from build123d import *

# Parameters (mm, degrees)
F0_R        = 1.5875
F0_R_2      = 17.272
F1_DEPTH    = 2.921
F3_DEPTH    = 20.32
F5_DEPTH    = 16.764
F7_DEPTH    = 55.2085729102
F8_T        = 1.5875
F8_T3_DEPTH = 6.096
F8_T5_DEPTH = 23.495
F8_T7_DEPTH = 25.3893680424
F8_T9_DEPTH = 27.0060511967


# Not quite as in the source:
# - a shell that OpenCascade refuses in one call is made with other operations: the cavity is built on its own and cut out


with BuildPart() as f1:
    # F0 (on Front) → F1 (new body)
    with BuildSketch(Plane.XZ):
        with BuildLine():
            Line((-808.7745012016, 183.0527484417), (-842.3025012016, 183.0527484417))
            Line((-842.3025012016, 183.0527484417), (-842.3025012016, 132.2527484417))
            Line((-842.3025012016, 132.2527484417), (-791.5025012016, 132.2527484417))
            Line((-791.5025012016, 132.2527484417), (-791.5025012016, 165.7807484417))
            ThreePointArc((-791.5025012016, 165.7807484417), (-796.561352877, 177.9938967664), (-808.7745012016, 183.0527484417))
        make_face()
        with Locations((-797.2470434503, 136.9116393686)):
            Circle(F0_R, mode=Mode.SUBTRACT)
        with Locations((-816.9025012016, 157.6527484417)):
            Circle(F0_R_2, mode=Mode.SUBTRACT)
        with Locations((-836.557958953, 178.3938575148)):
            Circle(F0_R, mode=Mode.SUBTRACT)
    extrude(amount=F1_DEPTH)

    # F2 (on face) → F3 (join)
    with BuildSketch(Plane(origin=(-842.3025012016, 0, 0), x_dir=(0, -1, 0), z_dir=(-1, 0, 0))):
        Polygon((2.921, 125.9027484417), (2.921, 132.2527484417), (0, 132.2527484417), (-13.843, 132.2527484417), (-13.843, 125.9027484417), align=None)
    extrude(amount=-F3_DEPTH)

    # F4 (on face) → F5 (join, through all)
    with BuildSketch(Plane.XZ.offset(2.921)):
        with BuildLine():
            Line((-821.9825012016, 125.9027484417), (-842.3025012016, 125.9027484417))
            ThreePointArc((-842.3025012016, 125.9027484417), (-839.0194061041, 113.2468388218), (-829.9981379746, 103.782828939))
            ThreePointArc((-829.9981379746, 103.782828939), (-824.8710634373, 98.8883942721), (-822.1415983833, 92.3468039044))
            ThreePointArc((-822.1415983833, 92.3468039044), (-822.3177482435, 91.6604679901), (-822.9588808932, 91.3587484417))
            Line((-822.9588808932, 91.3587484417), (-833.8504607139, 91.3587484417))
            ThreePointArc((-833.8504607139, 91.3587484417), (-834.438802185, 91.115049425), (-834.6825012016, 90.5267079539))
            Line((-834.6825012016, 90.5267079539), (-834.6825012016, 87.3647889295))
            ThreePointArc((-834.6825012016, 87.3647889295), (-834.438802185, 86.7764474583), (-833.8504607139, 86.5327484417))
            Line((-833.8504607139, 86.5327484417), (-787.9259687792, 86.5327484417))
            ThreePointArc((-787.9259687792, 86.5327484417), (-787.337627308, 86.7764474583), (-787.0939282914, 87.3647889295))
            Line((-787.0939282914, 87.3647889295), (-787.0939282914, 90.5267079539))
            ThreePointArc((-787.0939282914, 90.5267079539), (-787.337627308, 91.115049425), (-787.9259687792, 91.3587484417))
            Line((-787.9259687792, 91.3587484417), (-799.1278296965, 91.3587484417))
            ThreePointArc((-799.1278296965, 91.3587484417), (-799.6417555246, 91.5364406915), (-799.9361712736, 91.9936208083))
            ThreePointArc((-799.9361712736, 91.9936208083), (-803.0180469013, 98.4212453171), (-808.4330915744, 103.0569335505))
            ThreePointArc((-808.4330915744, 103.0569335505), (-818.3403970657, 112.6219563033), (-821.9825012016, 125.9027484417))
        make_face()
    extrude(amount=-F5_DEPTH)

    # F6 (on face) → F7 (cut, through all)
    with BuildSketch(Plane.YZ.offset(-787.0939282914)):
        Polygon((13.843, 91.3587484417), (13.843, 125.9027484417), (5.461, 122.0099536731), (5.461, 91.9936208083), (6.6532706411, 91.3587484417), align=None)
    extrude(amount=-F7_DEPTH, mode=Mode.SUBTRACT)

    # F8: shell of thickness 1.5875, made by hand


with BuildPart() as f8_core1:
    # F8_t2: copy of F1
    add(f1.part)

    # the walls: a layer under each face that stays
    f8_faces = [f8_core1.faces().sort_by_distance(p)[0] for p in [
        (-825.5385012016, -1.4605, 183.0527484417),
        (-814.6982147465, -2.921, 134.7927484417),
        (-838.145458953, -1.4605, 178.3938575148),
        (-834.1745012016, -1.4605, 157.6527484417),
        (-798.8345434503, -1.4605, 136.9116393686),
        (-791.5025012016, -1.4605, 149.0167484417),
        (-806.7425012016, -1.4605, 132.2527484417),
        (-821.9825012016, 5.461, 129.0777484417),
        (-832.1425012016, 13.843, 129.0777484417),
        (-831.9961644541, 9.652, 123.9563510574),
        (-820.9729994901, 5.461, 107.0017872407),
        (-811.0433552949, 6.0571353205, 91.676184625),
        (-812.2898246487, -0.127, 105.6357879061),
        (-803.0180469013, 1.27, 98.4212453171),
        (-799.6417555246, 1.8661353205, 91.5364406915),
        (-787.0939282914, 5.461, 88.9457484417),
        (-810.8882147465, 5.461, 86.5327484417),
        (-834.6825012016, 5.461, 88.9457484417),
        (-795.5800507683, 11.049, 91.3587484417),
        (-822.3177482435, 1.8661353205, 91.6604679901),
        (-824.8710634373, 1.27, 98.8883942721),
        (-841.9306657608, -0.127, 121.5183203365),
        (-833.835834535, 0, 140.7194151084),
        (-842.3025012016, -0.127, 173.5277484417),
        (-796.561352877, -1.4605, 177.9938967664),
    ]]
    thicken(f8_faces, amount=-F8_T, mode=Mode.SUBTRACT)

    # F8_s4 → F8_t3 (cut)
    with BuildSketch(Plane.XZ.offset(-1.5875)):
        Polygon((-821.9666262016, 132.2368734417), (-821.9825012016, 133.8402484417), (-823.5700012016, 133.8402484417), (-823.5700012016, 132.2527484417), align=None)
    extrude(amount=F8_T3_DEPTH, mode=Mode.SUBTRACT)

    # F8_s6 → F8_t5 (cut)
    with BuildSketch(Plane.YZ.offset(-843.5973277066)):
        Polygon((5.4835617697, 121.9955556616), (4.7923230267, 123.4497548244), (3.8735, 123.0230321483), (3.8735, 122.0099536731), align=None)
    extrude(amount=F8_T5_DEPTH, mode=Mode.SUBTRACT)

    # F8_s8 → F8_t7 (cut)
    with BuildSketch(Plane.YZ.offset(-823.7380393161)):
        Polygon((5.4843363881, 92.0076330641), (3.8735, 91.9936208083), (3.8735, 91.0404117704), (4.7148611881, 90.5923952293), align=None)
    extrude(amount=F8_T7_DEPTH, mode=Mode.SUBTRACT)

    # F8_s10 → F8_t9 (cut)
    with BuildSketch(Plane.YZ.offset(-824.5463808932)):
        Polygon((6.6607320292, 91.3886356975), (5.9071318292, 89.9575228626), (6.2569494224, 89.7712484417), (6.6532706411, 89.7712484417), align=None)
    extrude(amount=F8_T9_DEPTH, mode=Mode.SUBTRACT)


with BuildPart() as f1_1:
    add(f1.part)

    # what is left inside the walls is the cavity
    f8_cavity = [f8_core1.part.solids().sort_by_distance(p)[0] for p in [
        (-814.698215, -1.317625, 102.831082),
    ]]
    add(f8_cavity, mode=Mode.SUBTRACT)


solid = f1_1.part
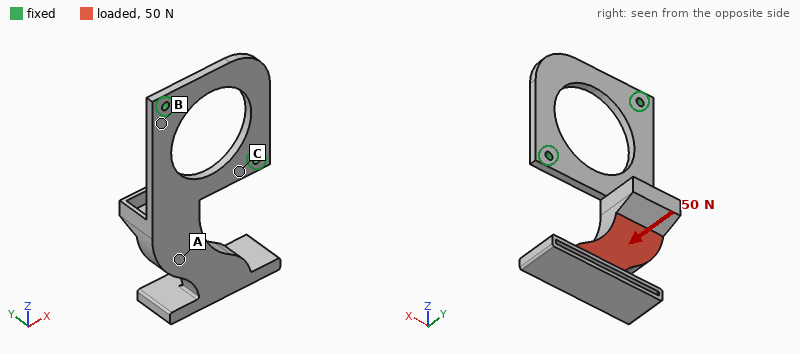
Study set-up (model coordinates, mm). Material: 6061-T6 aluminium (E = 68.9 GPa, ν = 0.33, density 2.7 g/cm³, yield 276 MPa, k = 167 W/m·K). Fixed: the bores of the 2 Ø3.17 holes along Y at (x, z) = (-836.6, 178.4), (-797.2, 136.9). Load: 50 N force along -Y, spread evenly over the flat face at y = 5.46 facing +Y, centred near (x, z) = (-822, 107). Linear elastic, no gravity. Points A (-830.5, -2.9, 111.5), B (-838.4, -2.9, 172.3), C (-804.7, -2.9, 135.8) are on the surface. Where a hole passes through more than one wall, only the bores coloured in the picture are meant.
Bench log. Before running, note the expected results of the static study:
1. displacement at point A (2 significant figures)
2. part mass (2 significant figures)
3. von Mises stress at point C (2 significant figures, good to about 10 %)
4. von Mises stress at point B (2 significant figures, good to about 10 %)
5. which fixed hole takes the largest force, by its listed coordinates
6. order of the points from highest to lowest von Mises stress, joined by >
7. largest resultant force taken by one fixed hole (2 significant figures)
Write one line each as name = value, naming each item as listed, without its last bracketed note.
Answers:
displacement at point A = 0.63 mm
part mass = 30 g
von Mises stress at point C = 75 MPa
von Mises stress at point B = 25 MPa
which fixed hole takes the largest force, by its listed coordinates = (-797.2, 136.9)
order of the points from highest to lowest von Mises stress, joined by > = C > B > A
largest resultant force taken by one fixed hole = 60 N
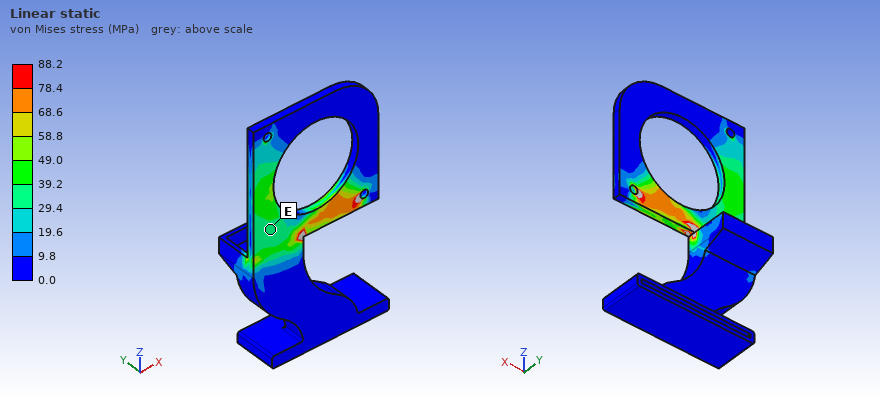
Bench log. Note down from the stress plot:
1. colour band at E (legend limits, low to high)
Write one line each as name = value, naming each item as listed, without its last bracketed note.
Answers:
colour band at E = 29.4 to 39.2 MPa
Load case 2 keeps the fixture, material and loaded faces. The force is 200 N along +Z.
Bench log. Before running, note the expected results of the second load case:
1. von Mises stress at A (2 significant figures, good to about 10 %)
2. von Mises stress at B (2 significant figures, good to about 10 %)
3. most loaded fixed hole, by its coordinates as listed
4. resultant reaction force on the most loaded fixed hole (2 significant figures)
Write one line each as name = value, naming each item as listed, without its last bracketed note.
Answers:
von Mises stress at A = 5.1 MPa
von Mises stress at B = 9.4 MPa
most loaded fixed hole, by its coordinates as listed = (-836.6, 178.4)
resultant reaction force on the most loaded fixed hole = 120 N
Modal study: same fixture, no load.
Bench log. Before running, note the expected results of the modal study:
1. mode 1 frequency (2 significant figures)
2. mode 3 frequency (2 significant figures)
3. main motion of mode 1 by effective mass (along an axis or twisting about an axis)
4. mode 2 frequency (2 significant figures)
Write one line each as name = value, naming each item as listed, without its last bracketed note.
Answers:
mode 1 frequency = 290 Hz
mode 3 frequency = 1600 Hz
main motion of mode 1 by effective mass = along Y
mode 2 frequency = 810 Hz
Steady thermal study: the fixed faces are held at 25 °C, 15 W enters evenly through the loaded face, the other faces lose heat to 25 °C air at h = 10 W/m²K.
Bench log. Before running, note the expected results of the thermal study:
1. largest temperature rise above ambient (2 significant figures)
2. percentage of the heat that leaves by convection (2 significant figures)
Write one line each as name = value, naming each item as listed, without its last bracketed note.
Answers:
largest temperature rise above ambient = 68 K
percentage of the heat that leaves by convection = 33 %
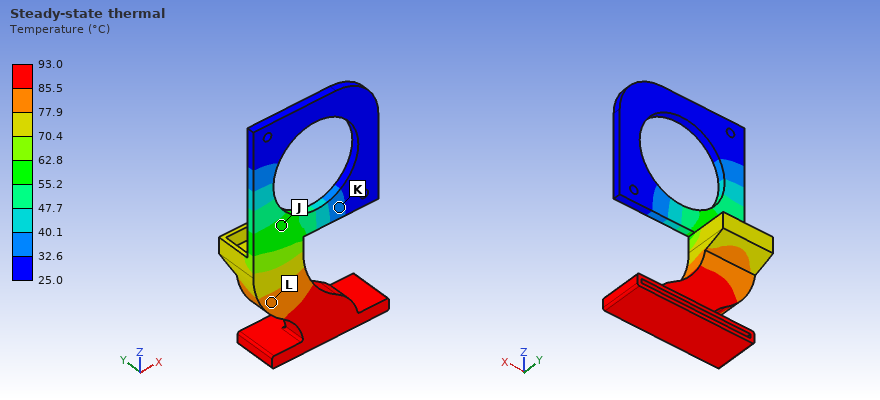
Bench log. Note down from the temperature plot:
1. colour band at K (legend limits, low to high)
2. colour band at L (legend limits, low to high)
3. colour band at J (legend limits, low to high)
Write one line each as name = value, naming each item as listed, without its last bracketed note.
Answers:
colour band at K = 32.6 to 40.1 °C
colour band at L = 77.9 to 85.5 °C
colour band at J = 55.2 to 62.8 °C
